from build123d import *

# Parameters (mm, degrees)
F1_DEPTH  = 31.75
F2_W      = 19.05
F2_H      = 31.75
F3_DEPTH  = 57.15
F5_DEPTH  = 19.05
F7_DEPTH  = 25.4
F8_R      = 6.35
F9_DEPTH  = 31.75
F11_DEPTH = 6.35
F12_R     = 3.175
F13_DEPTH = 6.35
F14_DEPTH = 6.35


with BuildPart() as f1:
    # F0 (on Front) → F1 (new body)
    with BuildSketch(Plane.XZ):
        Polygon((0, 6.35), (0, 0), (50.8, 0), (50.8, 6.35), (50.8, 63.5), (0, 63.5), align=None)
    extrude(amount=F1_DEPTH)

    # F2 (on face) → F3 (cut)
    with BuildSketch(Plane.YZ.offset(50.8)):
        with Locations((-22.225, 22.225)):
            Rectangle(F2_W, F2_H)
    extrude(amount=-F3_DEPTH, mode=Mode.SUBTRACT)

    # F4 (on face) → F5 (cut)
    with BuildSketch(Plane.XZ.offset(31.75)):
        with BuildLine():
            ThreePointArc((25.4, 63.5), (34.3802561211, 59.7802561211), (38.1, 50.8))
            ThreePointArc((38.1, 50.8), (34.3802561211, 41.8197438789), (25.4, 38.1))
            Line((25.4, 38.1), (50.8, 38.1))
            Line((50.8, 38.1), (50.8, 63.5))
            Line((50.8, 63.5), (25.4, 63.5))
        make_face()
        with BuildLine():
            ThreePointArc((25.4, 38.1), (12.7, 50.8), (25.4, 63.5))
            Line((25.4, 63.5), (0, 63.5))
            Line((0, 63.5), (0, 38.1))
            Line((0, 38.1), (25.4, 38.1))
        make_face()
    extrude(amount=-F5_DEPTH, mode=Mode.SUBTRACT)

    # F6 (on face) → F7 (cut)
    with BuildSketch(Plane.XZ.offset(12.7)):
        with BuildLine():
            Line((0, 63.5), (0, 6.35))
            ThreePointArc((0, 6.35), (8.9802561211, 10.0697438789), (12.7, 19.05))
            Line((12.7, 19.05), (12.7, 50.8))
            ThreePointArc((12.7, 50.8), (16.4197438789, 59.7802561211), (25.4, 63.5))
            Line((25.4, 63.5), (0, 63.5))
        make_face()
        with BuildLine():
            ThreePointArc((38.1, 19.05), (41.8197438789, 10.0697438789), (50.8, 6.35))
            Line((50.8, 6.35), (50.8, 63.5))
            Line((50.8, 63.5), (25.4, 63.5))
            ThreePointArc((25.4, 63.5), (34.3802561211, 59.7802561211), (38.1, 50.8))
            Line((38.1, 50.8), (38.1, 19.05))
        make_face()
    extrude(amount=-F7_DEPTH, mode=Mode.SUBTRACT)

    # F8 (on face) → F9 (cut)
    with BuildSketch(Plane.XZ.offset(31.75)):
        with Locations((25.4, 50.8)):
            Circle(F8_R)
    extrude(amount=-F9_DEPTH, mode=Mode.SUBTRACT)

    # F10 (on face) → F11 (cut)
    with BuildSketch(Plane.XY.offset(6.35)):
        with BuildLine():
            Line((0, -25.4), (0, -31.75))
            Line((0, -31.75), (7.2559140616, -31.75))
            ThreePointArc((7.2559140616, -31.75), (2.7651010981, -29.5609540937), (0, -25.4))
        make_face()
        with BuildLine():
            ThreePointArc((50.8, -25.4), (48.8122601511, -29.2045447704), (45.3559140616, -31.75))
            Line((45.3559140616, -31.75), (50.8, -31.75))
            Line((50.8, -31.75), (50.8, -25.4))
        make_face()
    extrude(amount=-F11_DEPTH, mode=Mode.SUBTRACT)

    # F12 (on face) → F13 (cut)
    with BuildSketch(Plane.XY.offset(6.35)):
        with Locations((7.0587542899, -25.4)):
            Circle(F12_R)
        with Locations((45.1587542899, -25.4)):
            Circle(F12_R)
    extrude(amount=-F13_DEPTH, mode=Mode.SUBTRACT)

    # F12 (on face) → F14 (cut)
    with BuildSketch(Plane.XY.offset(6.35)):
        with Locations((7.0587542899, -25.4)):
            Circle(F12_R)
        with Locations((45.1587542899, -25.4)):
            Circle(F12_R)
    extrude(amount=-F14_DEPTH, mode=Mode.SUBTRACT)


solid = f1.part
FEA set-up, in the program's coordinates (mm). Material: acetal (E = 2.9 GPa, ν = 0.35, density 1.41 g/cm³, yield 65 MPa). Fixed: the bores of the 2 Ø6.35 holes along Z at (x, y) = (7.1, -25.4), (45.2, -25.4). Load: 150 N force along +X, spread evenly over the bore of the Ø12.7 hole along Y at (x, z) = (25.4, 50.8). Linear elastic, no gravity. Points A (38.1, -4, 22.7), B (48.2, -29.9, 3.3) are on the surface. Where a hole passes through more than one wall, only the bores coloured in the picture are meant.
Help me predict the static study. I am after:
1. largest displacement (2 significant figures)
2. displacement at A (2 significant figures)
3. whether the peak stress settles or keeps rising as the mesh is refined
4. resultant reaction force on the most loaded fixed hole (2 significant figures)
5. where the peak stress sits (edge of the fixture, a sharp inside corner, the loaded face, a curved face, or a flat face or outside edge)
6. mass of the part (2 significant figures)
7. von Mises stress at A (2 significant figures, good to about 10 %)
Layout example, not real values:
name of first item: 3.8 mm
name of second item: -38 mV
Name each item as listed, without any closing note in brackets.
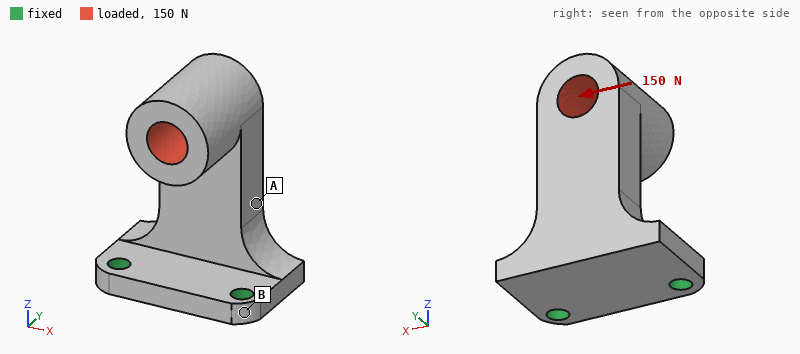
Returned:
largest displacement: 0.63 mm
displacement at A: 0.17 mm
whether the peak stress settles or keeps rising as the mesh is refined: keeps rising
resultant reaction force on the most loaded fixed hole: 210 N
where the peak stress sits: edge of the fixture
mass of the part: 48 g
von Mises stress at A: 3.3 MPa
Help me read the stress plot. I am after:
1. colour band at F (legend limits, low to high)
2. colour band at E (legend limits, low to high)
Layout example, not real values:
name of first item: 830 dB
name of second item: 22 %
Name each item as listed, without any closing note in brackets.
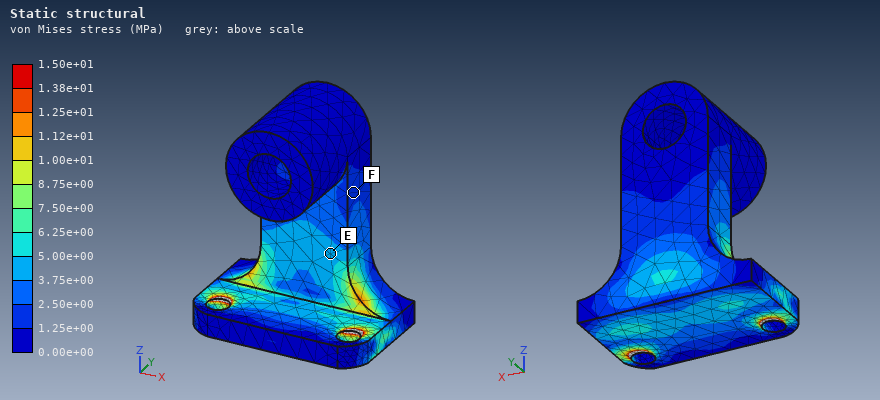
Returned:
colour band at F: 1.25e+00 to 2.50e+00 MPa
colour band at E: 3.75e+00 to 5.00e+00 MPa
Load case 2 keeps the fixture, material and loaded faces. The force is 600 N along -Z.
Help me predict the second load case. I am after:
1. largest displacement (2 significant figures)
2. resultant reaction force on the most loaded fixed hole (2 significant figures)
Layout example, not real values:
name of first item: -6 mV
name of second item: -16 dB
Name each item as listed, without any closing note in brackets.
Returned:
largest displacement: 0.63 mm
resultant reaction force on the most loaded fixed hole: 310 N
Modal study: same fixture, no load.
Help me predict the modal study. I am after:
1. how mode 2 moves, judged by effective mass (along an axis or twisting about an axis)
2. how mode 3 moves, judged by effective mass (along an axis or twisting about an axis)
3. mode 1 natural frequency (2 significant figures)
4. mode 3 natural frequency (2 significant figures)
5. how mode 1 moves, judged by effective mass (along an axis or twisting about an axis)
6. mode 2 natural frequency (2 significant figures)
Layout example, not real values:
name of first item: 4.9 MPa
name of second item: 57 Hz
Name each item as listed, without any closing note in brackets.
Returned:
how mode 2 moves, judged by effective mass: along X
how mode 3 moves, judged by effective mass: along Z
mode 1 natural frequency: 280 Hz
mode 3 natural frequency: 1200 Hz
how mode 1 moves, judged by effective mass: along Y
mode 2 natural frequency: 650 Hz
